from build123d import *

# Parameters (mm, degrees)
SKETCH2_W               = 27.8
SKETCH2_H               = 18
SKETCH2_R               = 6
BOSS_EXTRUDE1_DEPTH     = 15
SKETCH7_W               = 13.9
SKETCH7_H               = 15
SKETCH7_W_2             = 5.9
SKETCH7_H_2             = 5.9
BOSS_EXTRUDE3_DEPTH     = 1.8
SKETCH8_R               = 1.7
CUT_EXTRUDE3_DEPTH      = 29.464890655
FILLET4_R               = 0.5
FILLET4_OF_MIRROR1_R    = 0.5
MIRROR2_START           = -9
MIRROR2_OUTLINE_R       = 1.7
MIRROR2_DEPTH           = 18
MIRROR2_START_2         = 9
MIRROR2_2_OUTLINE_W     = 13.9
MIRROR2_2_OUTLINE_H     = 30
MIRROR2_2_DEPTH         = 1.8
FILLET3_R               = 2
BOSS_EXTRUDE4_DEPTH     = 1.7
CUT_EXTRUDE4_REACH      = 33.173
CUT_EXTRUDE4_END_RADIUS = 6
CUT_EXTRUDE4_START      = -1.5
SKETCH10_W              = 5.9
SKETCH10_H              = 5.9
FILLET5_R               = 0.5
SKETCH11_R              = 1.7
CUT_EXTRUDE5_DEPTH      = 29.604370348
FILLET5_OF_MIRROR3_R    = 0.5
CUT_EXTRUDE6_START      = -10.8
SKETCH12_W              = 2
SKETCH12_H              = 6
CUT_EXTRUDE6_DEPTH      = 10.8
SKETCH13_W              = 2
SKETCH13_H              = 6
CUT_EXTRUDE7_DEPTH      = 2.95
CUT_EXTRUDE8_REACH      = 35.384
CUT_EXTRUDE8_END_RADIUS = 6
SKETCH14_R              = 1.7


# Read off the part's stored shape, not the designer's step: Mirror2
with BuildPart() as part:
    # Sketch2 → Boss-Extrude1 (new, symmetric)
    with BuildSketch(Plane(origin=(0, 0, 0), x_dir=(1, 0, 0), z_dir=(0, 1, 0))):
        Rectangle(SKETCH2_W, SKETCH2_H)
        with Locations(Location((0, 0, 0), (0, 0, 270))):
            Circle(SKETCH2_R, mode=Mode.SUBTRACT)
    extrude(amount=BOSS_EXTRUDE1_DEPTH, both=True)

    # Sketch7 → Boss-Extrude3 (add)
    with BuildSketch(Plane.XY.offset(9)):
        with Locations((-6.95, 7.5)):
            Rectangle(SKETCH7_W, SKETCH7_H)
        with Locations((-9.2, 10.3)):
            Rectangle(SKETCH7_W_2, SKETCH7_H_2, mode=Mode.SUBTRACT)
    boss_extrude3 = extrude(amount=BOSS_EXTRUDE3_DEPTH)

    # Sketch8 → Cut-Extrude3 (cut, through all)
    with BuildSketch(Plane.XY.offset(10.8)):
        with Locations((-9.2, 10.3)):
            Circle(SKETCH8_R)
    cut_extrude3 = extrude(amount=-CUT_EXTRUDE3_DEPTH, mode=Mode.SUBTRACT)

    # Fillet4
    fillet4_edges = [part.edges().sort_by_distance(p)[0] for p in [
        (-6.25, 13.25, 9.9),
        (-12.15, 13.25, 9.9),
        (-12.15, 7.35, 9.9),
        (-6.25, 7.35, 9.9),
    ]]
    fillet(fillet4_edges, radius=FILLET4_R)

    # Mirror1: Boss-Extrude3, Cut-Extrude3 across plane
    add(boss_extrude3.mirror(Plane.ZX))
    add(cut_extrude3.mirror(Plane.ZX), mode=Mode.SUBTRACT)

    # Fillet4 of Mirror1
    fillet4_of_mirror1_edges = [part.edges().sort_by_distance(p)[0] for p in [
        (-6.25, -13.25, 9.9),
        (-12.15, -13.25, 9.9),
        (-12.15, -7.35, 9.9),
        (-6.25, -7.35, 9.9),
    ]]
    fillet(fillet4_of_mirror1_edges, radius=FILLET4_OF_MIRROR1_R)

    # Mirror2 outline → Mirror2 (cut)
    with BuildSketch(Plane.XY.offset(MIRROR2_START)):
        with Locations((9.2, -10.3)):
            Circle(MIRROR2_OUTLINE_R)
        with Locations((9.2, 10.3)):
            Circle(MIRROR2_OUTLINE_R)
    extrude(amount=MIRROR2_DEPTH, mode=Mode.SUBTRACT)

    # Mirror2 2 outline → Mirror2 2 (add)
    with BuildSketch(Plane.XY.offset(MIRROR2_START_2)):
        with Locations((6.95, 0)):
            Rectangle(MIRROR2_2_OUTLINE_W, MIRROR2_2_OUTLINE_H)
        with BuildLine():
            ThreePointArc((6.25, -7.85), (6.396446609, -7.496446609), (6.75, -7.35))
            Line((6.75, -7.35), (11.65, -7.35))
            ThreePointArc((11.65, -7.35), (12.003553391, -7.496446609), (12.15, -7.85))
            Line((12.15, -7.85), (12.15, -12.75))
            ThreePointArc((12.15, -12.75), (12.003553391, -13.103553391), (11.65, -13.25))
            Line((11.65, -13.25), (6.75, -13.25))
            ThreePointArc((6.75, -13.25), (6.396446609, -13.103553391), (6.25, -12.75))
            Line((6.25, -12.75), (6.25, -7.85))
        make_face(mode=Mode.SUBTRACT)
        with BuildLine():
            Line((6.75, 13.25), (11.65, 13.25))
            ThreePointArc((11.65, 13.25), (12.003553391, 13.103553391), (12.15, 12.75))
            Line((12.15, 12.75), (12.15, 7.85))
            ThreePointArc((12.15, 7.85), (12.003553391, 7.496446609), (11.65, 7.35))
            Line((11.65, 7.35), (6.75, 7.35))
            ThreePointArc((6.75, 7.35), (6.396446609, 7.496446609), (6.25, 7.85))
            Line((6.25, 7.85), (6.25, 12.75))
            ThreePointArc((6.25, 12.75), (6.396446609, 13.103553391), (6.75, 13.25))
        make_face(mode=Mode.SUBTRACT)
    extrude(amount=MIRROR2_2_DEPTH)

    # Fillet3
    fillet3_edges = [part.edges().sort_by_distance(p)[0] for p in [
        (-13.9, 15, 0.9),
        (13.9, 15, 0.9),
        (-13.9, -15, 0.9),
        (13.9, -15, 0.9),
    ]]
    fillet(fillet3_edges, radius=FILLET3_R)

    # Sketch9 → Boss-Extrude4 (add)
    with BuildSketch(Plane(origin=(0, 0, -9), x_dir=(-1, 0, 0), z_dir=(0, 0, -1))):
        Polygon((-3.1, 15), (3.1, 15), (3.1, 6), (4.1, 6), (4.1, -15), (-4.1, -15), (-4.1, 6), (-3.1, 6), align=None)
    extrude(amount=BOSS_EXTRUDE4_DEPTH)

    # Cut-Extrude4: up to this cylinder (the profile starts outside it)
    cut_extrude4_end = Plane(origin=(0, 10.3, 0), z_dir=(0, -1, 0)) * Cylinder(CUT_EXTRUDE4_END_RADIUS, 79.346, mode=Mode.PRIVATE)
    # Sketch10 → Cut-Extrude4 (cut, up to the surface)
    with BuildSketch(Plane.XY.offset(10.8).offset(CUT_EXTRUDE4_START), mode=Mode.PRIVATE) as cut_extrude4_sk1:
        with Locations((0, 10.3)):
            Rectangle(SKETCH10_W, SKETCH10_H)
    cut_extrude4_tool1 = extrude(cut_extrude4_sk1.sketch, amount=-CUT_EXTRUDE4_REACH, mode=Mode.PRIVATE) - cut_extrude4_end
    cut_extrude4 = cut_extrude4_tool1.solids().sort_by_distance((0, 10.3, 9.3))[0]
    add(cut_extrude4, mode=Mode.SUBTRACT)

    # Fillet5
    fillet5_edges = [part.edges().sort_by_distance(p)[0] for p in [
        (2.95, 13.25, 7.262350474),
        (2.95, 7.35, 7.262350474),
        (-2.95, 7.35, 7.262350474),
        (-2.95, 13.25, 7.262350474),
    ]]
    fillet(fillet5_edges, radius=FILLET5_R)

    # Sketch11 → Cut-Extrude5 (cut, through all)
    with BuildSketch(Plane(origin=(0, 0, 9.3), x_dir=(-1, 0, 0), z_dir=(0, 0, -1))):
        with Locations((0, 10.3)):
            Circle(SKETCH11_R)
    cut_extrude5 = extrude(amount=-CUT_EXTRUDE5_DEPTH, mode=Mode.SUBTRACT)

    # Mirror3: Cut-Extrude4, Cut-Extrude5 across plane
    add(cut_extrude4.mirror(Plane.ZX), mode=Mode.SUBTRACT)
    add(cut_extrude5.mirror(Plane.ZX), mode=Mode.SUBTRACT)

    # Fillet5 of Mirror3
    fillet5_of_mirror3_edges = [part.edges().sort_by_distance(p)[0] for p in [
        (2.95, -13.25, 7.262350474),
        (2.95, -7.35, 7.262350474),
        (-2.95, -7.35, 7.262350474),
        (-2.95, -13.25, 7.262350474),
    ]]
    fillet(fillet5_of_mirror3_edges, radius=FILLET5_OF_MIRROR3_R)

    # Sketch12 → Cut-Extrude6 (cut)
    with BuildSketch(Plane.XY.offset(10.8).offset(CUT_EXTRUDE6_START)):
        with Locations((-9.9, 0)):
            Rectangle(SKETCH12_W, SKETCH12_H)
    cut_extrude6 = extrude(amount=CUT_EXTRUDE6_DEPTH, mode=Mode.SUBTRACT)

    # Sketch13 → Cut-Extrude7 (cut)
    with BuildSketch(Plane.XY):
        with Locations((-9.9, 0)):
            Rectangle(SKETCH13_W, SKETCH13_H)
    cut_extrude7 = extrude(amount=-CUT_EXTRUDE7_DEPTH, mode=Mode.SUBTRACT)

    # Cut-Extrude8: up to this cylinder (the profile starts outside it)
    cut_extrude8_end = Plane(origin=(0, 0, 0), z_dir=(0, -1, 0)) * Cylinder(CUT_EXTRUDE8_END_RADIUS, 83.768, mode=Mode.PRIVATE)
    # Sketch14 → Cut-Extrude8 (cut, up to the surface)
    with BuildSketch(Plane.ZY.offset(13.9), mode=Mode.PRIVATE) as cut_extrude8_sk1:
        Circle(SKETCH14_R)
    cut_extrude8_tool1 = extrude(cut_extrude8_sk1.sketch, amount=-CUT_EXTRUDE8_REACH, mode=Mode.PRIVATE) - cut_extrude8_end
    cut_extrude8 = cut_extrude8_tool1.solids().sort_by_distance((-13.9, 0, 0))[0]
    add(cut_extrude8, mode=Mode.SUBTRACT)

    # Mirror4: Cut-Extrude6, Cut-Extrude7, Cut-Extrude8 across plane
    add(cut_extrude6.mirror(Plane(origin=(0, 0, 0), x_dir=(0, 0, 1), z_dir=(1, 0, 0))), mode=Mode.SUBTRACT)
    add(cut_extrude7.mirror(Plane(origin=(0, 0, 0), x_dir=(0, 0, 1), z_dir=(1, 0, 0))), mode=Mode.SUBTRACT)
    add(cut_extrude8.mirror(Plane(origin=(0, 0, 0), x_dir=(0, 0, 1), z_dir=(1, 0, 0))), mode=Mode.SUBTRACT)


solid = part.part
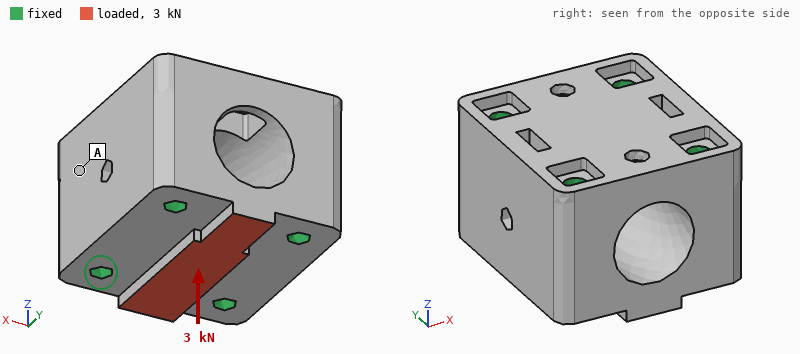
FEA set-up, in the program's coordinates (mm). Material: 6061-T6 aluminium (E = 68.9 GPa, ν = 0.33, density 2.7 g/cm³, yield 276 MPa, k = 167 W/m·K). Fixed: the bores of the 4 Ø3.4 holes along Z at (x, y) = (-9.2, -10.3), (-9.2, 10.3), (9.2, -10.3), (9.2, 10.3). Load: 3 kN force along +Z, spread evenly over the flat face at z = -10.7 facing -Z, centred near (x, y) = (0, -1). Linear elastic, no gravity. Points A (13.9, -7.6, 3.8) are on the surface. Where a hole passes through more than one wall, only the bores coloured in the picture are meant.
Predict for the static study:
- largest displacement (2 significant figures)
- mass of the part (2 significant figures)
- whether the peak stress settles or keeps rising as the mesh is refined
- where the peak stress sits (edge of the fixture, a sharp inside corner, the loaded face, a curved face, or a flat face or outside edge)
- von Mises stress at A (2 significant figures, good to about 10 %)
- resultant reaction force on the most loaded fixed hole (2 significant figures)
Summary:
4.3 µm
32 g
keeps rising
edge of the fixture
3.4 MPa
950 N
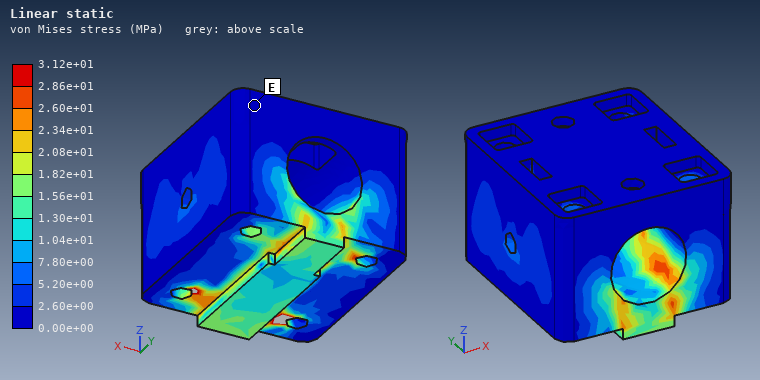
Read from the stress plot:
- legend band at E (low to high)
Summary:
0.00e+00 to 2.60e+00 MPa
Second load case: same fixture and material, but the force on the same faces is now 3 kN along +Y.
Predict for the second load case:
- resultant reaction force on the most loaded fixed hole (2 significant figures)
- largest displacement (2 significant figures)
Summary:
920 N
8.7 µm
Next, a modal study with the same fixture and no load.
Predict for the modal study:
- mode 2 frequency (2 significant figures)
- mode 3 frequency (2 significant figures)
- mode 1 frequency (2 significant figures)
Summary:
62 kHz
69 kHz
62 kHz
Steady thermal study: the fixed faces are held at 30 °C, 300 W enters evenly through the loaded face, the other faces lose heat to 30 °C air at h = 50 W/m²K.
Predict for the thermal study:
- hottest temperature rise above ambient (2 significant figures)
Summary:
68 K
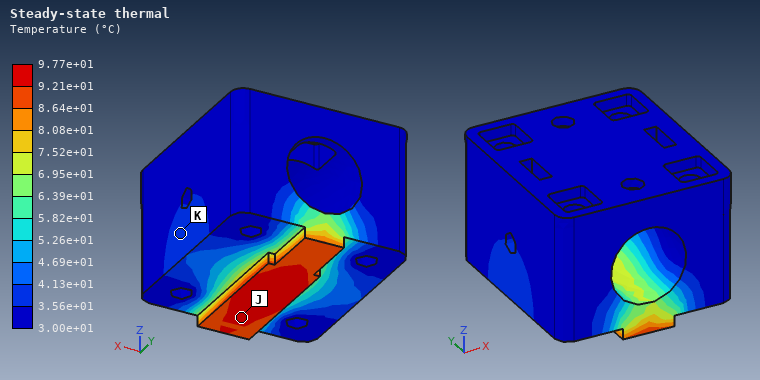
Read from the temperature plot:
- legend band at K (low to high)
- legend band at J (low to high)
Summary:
3.56e+01 to 4.13e+01 °C
9.21e+01 to 9.77e+01 °C
